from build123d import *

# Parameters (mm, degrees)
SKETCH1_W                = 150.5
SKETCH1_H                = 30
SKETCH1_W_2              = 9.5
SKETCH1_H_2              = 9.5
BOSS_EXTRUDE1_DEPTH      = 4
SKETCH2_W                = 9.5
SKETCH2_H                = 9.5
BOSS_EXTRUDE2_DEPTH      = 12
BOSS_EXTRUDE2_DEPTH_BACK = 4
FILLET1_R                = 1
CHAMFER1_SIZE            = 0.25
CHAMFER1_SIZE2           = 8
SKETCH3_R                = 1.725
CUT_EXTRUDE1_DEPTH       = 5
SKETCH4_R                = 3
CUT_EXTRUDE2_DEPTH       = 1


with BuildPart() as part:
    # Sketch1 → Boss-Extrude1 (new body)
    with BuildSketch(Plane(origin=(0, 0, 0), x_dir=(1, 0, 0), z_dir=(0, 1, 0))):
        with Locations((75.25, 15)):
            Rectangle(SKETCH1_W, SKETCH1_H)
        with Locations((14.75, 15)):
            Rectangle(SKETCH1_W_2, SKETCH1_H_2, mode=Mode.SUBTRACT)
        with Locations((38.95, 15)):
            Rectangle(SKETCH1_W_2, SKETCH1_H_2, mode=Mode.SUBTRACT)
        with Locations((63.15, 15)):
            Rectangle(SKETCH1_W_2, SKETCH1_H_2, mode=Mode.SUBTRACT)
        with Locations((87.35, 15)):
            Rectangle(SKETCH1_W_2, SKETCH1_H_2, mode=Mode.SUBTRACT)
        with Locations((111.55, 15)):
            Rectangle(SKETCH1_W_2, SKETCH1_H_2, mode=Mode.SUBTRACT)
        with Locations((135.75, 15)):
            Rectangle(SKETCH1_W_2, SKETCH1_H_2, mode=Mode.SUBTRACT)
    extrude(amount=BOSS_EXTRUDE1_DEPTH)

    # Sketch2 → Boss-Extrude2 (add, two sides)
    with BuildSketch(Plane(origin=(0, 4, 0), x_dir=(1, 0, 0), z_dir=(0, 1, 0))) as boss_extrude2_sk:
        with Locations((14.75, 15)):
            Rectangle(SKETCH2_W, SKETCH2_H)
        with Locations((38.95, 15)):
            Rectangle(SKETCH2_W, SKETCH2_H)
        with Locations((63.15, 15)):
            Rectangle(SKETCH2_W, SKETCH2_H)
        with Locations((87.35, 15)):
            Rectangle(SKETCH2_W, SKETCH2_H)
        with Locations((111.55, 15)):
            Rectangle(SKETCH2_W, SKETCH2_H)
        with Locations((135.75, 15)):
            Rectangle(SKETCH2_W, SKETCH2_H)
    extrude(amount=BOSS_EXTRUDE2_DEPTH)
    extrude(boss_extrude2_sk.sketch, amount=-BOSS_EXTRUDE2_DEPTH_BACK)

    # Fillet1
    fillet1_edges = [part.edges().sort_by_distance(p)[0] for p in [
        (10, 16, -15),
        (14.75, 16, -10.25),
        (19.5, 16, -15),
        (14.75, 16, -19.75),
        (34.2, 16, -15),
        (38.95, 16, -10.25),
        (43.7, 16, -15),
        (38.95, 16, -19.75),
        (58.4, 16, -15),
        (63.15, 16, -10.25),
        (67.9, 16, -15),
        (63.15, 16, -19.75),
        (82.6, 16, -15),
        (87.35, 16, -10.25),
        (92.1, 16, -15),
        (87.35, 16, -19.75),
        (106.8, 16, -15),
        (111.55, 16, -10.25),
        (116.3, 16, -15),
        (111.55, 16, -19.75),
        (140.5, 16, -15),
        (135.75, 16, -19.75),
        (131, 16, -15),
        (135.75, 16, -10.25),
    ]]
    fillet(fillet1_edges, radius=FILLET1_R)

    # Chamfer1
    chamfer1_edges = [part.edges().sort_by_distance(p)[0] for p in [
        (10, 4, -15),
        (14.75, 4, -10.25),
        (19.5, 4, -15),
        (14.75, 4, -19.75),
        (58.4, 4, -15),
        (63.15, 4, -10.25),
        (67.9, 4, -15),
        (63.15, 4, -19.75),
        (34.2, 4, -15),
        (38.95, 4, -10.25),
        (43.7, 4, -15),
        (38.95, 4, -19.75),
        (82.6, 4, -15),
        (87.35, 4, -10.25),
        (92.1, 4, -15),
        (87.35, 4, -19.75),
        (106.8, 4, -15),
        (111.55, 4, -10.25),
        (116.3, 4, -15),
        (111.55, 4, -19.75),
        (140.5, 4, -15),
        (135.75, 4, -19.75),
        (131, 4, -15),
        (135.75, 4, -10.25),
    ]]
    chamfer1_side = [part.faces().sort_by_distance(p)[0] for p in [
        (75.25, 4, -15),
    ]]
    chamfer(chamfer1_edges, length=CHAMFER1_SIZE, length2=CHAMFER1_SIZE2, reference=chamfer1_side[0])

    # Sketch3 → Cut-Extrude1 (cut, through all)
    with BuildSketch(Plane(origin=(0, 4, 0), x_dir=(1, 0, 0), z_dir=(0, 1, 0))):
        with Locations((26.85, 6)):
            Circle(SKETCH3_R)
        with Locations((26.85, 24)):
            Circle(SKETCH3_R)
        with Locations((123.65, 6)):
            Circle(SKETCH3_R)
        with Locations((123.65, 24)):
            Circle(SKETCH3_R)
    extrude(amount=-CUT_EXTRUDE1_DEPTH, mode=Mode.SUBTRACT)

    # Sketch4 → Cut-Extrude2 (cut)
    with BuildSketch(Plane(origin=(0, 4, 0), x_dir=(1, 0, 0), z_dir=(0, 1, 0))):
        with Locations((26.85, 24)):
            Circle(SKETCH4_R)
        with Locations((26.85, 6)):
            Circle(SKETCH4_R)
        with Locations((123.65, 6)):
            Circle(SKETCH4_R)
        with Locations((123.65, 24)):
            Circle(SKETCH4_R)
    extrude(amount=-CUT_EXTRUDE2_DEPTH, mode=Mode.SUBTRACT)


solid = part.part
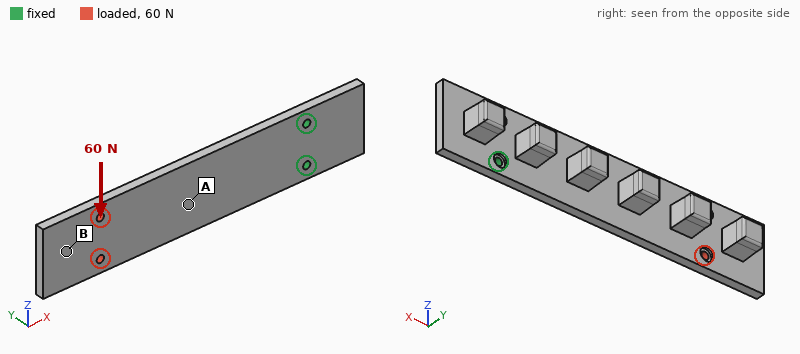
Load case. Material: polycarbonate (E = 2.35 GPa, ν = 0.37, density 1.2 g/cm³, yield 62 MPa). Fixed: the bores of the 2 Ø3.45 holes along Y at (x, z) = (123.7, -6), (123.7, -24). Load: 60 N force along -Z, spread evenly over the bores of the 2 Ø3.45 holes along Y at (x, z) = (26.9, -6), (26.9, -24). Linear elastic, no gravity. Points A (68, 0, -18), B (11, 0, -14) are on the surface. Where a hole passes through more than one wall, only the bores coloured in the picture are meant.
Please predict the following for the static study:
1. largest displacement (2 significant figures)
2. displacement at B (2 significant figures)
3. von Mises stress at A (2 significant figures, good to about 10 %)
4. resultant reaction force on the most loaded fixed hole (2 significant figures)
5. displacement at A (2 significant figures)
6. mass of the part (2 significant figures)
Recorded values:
1.4 mm
1.2 mm
1.8 MPa
300 N
0.44 mm
29 g
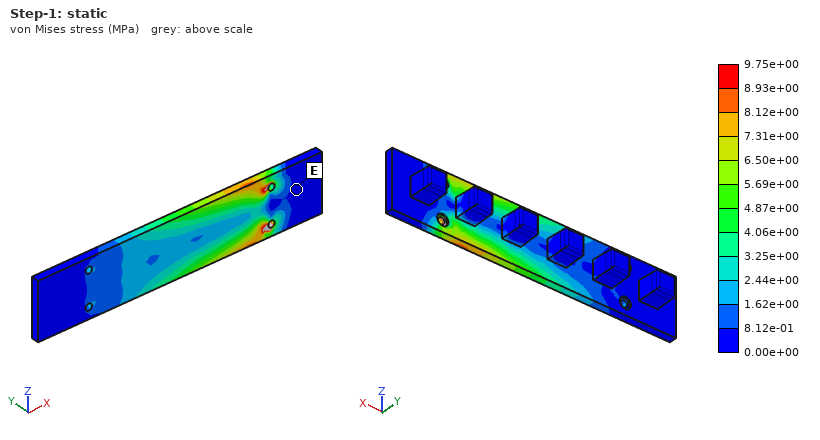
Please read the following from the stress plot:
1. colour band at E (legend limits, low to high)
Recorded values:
0.00e+00 to 8.12e-01 MPa
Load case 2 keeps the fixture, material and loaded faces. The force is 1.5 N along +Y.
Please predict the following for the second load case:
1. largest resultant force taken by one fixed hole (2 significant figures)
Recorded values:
1.0 N
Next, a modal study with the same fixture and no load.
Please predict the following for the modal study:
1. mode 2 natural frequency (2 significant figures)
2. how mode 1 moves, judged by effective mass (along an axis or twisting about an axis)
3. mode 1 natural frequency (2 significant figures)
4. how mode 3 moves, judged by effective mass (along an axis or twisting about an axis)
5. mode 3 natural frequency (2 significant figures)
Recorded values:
330 Hz
along Y
54 Hz
along Z
350 Hz
